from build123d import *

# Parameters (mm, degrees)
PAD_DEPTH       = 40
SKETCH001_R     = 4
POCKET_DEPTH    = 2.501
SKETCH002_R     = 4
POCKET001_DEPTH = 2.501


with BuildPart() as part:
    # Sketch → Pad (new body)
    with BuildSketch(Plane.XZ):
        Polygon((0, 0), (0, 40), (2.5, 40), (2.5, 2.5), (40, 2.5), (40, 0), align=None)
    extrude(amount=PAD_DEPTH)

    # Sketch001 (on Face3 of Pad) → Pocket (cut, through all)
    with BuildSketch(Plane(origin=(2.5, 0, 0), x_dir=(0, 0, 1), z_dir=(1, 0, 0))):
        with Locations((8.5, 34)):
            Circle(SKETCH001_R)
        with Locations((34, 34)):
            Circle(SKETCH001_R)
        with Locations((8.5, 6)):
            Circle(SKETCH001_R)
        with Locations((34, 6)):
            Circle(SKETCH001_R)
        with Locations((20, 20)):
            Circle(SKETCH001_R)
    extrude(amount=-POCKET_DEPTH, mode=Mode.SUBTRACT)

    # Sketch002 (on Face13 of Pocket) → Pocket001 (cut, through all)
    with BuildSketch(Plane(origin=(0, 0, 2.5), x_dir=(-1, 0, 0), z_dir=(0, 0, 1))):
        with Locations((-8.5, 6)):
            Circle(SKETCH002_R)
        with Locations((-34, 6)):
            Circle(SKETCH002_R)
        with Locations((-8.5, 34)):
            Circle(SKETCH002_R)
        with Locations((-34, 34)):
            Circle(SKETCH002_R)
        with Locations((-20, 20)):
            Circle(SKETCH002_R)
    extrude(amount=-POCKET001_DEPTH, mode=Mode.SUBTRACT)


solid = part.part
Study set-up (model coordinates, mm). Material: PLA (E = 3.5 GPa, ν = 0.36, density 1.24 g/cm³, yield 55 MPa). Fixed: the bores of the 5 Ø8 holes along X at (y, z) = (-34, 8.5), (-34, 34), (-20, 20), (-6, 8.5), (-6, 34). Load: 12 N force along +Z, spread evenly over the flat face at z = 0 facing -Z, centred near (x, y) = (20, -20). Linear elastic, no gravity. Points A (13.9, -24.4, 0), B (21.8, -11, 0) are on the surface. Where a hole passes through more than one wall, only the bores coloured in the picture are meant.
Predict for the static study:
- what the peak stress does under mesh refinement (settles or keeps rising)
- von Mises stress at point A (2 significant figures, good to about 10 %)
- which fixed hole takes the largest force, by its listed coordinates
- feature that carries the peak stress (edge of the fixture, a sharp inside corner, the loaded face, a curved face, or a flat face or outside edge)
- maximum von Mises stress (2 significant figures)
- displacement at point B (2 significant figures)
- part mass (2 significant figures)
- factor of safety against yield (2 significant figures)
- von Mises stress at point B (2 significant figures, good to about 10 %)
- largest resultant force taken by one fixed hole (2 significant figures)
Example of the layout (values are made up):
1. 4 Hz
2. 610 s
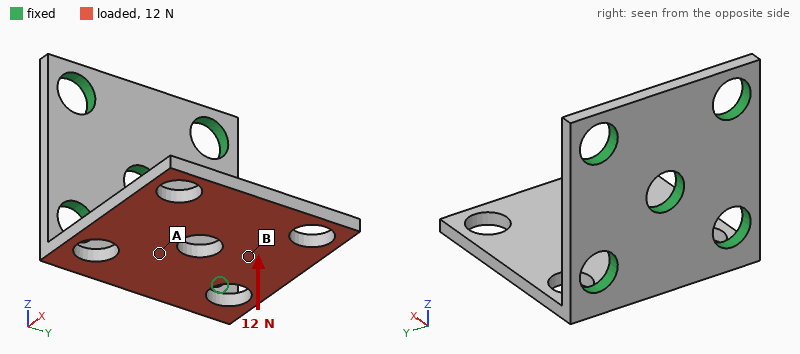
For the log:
1. settles
2. 3.0 MPa
3. (-20, 20)
4. the loaded face
5. 10 MPa
6. 0.33 mm
7. 8.1 g
8. 5.2
9. 1.4 MPa
10. 6.5 N
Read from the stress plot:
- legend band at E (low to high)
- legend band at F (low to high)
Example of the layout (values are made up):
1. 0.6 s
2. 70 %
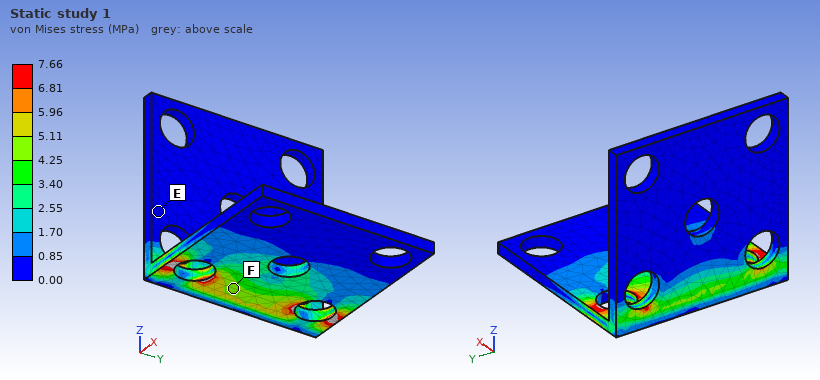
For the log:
1. 0.00 to 0.85 MPa
2. 4.25 to 5.11 MPa
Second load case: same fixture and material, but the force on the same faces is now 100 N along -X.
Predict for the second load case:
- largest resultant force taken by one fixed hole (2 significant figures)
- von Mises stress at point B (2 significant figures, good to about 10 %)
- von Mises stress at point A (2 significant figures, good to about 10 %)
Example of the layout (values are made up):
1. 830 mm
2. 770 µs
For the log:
1. 54 N
2. 2.1 MPa
3. 3.0 MPa
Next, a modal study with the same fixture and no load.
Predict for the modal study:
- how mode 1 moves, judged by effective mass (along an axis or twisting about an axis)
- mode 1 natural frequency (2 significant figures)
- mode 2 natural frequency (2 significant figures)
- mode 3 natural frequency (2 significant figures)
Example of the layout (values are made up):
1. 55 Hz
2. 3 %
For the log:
1. along Z
2. 380 Hz
3. 990 Hz
4. 2300 Hz
